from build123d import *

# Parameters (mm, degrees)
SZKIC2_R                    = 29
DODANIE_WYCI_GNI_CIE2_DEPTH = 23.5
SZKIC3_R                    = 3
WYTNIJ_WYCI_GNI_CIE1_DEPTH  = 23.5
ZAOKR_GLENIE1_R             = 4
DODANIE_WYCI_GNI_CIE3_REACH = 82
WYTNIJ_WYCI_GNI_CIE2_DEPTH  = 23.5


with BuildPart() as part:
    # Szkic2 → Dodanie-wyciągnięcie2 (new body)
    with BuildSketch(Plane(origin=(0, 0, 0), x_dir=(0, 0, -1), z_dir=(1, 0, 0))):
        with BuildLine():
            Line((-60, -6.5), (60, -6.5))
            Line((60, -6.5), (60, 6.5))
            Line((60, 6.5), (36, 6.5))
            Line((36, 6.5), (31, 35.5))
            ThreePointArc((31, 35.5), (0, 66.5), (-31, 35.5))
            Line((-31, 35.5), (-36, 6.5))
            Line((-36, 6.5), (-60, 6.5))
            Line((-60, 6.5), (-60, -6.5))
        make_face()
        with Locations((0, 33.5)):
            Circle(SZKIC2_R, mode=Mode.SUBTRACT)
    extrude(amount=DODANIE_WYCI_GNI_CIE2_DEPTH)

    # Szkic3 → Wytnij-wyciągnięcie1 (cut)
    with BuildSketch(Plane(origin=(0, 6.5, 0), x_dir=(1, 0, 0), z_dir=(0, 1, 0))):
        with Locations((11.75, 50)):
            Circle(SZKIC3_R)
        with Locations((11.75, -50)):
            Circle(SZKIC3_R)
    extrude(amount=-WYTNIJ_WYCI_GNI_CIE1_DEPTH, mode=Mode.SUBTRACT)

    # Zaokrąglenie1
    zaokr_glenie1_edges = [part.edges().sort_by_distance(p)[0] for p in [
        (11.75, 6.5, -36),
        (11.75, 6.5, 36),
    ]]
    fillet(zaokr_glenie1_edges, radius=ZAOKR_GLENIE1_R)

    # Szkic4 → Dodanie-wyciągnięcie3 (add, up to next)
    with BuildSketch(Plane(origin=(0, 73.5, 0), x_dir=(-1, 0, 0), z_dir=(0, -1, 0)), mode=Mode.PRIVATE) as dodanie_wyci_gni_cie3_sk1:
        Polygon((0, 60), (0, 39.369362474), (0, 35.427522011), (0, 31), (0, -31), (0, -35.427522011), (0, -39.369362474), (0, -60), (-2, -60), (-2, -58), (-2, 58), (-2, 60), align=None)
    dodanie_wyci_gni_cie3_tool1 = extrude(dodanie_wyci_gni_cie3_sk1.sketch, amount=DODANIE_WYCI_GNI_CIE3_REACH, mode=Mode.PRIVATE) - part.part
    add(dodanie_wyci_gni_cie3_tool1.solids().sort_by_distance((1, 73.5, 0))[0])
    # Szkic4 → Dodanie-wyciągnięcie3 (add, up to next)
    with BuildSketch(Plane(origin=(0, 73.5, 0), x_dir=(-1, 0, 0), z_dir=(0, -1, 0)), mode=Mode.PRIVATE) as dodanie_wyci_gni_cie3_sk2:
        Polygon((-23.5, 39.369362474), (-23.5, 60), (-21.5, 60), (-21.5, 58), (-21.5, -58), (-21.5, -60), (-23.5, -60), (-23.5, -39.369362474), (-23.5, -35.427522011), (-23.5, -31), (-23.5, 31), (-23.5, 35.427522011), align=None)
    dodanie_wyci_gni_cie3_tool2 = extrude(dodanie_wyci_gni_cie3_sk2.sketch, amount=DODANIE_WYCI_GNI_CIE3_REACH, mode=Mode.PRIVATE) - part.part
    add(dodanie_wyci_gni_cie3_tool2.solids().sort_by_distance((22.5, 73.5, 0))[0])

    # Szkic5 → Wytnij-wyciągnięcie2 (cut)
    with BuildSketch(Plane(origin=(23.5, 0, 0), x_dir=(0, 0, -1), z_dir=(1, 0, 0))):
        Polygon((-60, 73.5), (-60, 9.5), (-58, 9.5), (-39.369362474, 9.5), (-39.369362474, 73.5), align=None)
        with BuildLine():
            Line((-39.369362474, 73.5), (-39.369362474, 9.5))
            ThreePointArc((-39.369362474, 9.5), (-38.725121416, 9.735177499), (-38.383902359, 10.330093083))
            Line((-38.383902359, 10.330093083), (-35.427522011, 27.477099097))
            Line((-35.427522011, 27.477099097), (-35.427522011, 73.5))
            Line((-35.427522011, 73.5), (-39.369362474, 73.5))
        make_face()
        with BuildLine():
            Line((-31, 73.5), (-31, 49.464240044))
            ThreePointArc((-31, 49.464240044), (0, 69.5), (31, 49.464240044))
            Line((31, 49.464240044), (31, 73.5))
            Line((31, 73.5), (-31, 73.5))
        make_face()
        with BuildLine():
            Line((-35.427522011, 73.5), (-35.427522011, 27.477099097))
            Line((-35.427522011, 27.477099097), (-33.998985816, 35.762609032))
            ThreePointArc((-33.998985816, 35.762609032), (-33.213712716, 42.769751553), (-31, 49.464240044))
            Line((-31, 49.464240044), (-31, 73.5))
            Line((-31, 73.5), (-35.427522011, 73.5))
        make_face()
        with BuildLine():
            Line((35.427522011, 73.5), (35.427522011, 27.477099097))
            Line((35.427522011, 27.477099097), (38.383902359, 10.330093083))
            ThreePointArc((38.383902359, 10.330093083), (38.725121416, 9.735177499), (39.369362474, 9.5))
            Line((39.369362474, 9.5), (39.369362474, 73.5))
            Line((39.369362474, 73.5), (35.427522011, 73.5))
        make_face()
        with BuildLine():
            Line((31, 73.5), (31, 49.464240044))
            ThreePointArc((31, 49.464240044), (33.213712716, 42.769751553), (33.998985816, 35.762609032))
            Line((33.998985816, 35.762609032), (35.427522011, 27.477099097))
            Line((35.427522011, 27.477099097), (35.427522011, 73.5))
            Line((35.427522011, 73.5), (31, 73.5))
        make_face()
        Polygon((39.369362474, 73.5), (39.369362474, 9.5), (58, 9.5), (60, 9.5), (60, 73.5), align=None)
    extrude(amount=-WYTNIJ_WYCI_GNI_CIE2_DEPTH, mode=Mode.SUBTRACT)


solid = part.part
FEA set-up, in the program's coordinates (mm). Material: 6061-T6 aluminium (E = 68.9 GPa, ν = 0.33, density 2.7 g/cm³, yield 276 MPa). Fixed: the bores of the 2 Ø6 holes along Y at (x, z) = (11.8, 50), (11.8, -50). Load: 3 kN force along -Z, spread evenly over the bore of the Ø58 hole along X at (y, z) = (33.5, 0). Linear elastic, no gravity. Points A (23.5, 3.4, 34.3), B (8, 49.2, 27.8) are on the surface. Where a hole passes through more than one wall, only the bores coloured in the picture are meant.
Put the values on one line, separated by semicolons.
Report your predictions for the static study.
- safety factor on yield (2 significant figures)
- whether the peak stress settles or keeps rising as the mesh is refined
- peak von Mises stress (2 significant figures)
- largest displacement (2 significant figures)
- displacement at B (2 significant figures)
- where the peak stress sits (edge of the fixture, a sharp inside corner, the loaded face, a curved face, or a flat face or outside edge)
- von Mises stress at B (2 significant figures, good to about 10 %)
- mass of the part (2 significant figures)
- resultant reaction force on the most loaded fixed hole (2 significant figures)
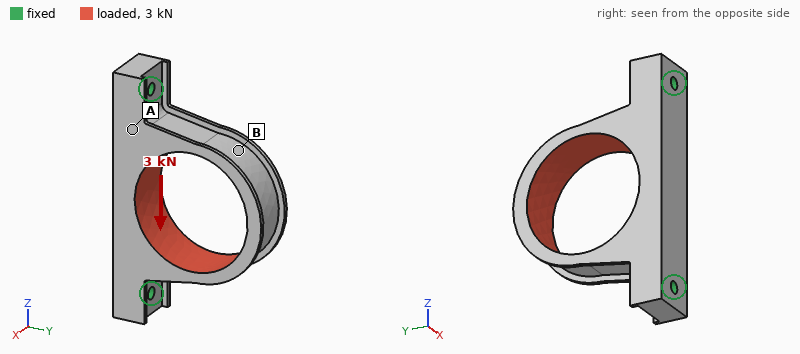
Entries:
1.8; settles; 150 MPa; 0.24 mm; 0.21 mm; a flat face or outside edge; 46 MPa; 160 g; 1.8 kN
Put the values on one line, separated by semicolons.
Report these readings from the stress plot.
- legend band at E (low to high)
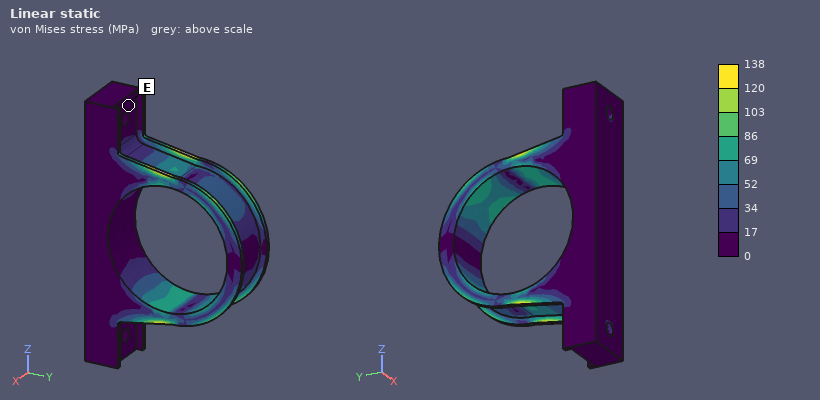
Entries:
0 to 17 MPa
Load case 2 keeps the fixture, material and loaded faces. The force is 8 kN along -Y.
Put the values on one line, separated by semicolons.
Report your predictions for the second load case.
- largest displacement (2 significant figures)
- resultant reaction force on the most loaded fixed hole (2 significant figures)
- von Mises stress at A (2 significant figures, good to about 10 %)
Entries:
84 µm; 4.0 kN; 22 MPa
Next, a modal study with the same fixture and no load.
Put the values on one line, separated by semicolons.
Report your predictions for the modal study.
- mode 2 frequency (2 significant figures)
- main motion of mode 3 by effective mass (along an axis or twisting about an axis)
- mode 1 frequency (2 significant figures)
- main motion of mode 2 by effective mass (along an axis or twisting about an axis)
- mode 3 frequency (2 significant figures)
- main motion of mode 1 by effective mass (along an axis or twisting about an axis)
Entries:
2700 Hz; along Y; 2500 Hz; along Z; 4900 Hz; along X
